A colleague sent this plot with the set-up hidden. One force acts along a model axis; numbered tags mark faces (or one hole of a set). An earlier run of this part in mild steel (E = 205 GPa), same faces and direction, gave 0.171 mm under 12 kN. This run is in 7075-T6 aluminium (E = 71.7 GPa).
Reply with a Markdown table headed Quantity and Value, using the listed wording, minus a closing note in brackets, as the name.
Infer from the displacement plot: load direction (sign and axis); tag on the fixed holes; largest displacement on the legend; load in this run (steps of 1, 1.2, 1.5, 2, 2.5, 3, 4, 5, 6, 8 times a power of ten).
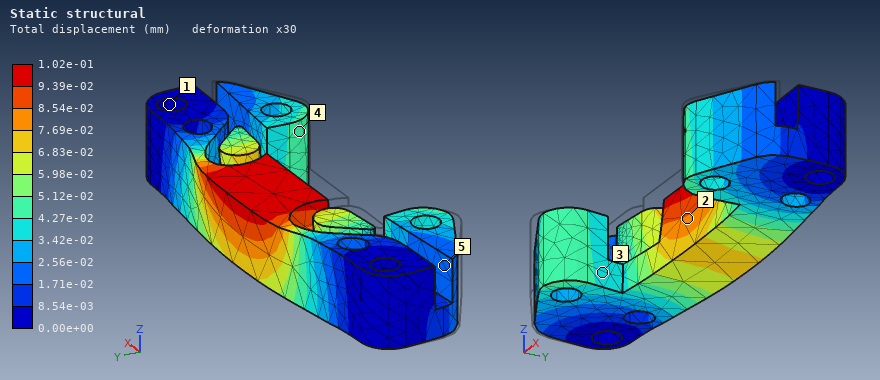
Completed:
| Quantity | Value |
|---|---|
| load direction | +Y |
| tag on the fixed holes | 1 |
| largest displacement on the legend | 1.02e-01 mm |
| load in this run | 2.5 kN |
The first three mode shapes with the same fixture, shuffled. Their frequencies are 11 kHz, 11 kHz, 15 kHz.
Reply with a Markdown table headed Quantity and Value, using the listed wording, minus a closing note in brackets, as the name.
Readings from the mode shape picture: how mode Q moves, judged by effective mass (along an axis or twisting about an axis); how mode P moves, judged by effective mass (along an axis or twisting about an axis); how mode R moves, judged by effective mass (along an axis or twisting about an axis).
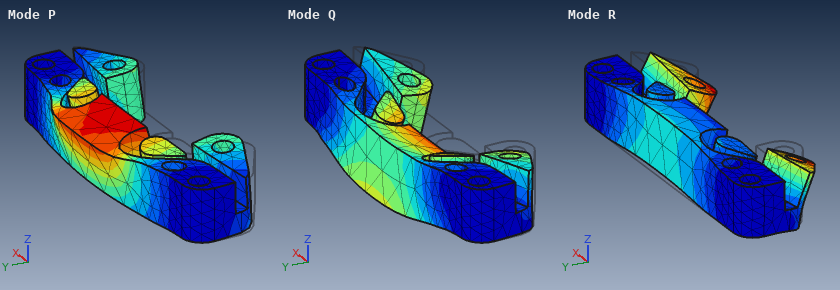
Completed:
| Quantity | Value |
|---|---|
| how mode Q moves, judged by effective mass | along Z |
| how mode P moves, judged by effective mass | along Y |
| how mode R moves, judged by effective mass | twisting about X |
